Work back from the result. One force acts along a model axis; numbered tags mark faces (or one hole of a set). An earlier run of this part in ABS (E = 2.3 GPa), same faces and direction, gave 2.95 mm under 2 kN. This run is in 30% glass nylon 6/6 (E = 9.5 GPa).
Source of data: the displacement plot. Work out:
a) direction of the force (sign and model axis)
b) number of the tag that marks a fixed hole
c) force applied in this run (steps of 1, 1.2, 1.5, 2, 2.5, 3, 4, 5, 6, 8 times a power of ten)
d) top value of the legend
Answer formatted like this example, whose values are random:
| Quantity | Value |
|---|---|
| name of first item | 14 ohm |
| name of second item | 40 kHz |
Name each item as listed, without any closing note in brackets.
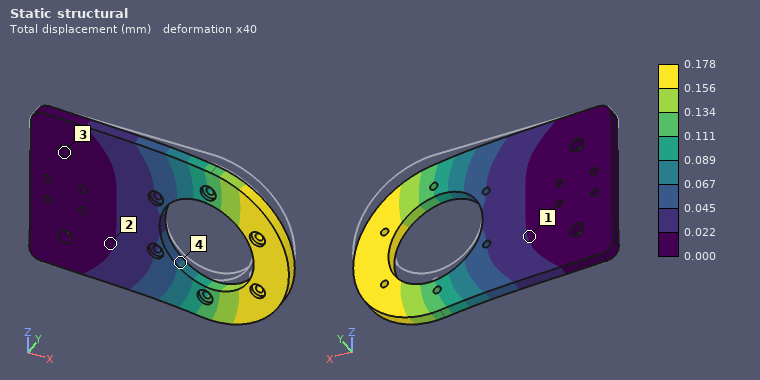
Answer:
| Quantity | Value |
|---|---|
| direction of the force | -Z |
| number of the tag that marks a fixed hole | 3 |
| force applied in this run | 500 N |
| top value of the legend | 0.178 mm |
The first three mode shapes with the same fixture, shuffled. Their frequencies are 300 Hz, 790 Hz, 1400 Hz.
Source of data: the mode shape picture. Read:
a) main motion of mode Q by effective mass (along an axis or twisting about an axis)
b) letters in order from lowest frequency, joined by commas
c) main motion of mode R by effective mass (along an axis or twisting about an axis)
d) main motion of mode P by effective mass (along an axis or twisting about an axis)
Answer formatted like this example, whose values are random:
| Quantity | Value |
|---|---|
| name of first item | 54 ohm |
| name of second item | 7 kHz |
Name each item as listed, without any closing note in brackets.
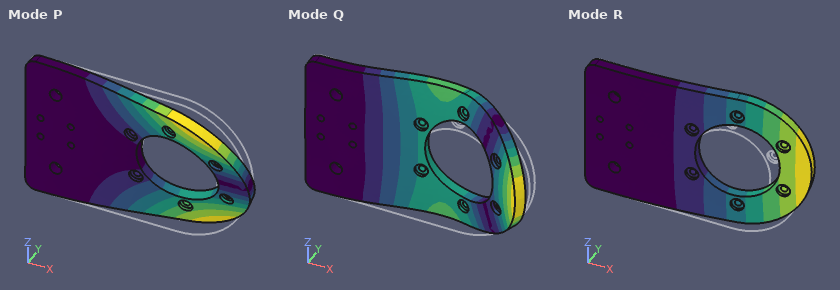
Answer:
| Quantity | Value |
|---|---|
| main motion of mode Q by effective mass | along Y |
| letters in order from lowest frequency, joined by commas | R, P, Q |
| main motion of mode R by effective mass | along Y |
| main motion of mode P by effective mass | twisting about X |
